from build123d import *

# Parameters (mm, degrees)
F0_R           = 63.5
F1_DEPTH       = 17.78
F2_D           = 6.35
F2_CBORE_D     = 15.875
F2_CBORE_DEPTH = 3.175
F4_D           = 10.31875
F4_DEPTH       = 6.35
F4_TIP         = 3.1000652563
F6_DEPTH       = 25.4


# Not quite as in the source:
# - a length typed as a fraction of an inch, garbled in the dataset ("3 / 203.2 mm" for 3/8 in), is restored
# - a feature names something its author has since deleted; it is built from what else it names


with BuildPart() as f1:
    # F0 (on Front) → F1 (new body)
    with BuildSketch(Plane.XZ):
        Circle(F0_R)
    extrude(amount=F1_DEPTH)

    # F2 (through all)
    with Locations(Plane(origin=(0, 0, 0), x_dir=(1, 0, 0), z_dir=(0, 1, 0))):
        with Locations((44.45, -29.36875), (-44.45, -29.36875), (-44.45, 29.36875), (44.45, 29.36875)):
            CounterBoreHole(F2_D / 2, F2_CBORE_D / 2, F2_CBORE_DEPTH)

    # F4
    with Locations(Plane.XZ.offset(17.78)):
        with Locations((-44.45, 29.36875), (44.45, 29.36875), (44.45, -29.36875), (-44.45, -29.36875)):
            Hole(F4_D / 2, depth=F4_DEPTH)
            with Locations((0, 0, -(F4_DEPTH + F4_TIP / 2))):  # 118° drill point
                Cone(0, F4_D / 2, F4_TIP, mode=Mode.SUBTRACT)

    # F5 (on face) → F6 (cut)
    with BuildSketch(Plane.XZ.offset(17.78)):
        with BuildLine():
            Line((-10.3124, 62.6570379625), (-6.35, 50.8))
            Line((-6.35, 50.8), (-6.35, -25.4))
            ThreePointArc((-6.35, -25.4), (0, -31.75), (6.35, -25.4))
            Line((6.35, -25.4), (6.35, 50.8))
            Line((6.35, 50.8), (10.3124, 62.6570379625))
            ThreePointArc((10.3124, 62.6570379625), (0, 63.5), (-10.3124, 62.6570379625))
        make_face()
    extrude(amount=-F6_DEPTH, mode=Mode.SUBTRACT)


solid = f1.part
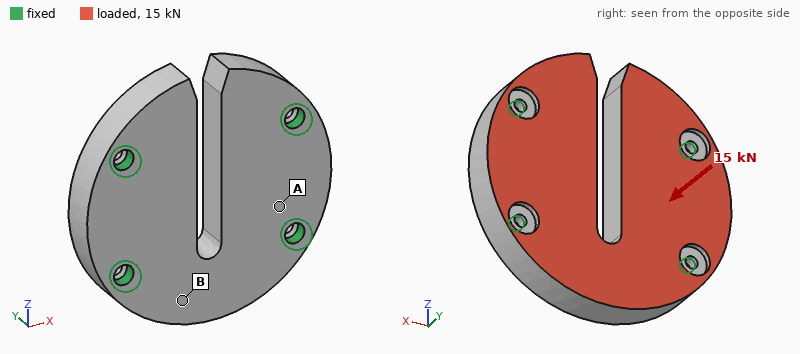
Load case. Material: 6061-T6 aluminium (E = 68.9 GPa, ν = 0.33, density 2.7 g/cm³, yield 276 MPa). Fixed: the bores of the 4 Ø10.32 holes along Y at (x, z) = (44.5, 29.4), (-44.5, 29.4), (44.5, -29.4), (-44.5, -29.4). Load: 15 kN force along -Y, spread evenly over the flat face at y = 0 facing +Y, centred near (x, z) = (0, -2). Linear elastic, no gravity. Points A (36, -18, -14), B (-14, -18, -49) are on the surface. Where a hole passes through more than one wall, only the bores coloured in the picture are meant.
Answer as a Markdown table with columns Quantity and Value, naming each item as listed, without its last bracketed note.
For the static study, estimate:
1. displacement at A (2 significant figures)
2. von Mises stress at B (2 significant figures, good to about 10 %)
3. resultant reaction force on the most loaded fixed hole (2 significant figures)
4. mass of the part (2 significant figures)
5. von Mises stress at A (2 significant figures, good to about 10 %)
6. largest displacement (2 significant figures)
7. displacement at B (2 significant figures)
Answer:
| Quantity | Value |
|---|---|
| displacement at A | 9.6 µm |
| von Mises stress at B | 15 MPa |
| resultant reaction force on the most loaded fixed hole | 4.4 kN |
| mass of the part | 530 g |
| von Mises stress at A | 6.8 MPa |
| largest displacement | 51 µm |
| displacement at B | 27 µm |
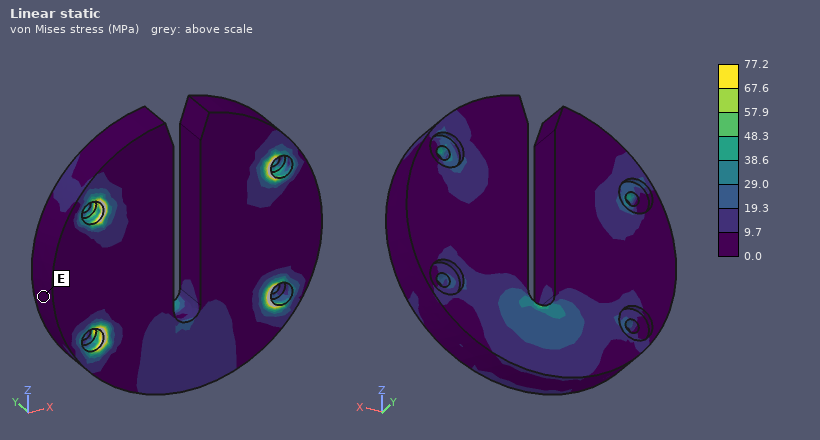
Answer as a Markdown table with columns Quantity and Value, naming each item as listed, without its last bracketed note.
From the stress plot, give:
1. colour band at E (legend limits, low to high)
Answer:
| Quantity | Value |
|---|---|
| colour band at E | 0.0 to 9.7 MPa |
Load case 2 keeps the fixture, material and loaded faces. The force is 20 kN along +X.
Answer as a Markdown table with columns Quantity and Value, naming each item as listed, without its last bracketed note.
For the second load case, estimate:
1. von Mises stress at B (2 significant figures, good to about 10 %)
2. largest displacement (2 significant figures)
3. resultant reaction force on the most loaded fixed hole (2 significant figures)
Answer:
| Quantity | Value |
|---|---|
| von Mises stress at B | 7.9 MPa |
| largest displacement | 49 µm |
| resultant reaction force on the most loaded fixed hole | 5.7 kN |
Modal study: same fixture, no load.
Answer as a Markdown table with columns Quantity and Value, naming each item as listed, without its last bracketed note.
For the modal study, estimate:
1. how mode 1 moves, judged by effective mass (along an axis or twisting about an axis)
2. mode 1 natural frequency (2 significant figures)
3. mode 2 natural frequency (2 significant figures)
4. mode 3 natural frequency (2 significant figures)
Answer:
| Quantity | Value |
|---|---|
| how mode 1 moves, judged by effective mass | along Y |
| mode 1 natural frequency | 4800 Hz |
| mode 2 natural frequency | 5300 Hz |
| mode 3 natural frequency | 6100 Hz |
